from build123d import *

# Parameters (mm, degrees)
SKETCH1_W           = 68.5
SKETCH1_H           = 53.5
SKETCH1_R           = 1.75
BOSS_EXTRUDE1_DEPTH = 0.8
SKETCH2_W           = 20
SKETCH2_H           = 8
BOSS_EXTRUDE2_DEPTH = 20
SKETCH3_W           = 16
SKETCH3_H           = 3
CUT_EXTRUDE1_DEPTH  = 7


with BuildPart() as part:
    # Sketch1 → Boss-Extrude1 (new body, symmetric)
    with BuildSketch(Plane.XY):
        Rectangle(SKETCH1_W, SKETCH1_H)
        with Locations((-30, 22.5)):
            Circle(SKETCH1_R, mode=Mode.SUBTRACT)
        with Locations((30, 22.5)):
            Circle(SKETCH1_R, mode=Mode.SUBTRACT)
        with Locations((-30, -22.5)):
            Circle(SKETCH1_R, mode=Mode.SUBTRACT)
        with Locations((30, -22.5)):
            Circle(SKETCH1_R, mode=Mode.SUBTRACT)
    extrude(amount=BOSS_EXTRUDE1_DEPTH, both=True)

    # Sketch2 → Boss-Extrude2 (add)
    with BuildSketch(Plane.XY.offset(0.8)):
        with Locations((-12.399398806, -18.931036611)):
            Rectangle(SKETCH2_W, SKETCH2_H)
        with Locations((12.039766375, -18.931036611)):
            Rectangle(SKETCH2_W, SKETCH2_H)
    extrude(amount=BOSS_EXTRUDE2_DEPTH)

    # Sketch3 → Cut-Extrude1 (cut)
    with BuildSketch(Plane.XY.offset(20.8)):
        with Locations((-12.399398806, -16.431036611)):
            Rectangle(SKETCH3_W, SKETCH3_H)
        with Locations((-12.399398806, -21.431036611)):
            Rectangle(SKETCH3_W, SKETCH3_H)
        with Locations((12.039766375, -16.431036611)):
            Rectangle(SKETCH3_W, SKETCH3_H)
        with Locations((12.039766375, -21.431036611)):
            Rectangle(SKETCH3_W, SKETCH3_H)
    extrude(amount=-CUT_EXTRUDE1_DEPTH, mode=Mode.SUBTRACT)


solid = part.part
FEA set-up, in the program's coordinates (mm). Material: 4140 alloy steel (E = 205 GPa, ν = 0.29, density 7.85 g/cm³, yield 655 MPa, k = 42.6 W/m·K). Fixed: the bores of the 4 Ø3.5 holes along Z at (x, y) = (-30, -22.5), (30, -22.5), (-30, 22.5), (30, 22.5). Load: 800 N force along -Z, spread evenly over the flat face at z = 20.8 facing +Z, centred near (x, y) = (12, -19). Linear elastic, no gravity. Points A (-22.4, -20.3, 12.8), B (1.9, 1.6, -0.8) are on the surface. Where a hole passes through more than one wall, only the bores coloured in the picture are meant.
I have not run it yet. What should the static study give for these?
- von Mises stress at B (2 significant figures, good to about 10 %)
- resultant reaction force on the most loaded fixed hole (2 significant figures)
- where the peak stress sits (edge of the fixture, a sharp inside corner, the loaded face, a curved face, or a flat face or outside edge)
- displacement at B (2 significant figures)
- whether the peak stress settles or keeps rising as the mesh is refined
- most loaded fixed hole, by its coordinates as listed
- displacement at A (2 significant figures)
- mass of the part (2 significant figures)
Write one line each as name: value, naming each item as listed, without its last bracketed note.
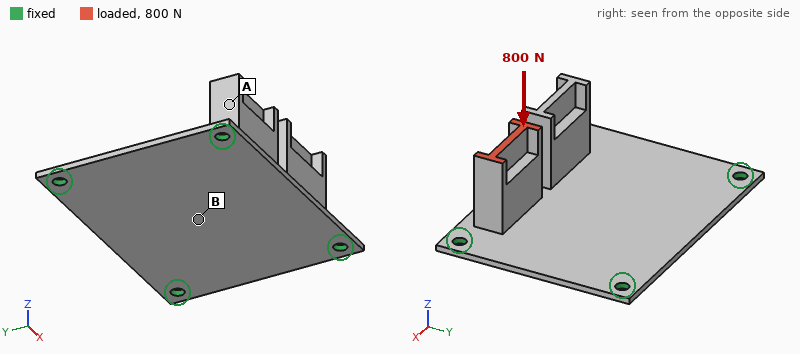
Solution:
von Mises stress at B: 80 MPa
resultant reaction force on the most loaded fixed hole: 590 N
where the peak stress sits: edge of the fixture
displacement at B: 0.13 mm
whether the peak stress settles or keeps rising as the mesh is refined: keeps rising
most loaded fixed hole, by its coordinates as listed: (30, -22.5)
displacement at A: 0.11 mm
mass of the part: 85 g
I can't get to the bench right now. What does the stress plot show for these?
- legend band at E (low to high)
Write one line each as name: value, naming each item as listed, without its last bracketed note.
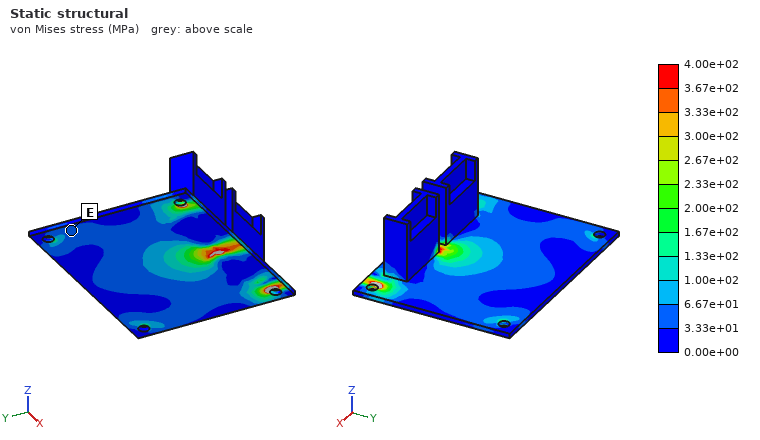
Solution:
legend band at E: 3.33e+01 to 6.67e+01 MPa
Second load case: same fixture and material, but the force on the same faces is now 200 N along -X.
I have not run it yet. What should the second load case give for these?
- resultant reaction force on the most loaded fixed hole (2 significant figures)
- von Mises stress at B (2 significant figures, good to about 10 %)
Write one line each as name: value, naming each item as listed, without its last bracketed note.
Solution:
resultant reaction force on the most loaded fixed hole: 120 N
von Mises stress at B: 31 MPa
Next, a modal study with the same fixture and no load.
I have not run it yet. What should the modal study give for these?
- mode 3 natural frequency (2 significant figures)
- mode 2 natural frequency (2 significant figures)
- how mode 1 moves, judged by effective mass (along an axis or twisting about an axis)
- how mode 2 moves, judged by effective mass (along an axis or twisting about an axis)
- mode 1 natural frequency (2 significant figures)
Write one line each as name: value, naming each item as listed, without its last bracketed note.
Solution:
mode 3 natural frequency: 3000 Hz
mode 2 natural frequency: 2000 Hz
how mode 1 moves, judged by effective mass: along Z
how mode 2 moves, judged by effective mass: along Y
mode 1 natural frequency: 1400 Hz
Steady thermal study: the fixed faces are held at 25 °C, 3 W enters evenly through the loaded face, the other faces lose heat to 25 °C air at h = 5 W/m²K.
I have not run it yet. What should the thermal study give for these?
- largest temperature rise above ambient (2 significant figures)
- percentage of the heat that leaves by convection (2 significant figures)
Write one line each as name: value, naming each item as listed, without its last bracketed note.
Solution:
largest temperature rise above ambient: 29 K
percentage of the heat that leaves by convection: 13 %
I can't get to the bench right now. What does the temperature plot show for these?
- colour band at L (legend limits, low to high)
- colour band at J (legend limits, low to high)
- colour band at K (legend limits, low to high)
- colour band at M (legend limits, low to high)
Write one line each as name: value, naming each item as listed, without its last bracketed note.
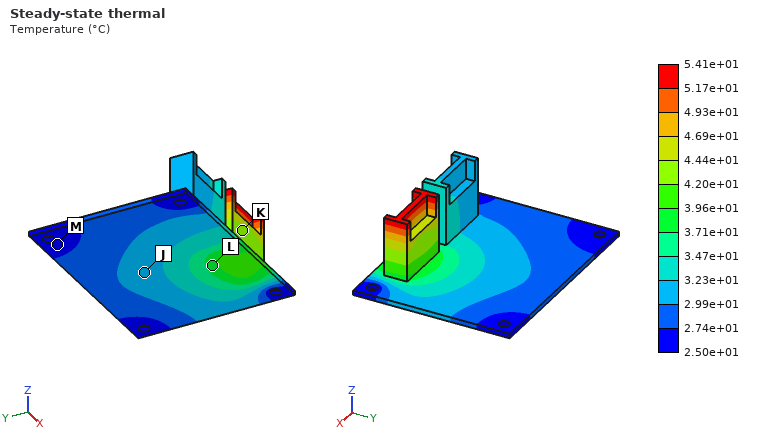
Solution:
colour band at L: 3.71e+01 to 3.96e+01 °C
colour band at J: 2.99e+01 to 3.23e+01 °C
colour band at K: 4.20e+01 to 4.44e+01 °C
colour band at M: 2.50e+01 to 2.74e+01 °C
